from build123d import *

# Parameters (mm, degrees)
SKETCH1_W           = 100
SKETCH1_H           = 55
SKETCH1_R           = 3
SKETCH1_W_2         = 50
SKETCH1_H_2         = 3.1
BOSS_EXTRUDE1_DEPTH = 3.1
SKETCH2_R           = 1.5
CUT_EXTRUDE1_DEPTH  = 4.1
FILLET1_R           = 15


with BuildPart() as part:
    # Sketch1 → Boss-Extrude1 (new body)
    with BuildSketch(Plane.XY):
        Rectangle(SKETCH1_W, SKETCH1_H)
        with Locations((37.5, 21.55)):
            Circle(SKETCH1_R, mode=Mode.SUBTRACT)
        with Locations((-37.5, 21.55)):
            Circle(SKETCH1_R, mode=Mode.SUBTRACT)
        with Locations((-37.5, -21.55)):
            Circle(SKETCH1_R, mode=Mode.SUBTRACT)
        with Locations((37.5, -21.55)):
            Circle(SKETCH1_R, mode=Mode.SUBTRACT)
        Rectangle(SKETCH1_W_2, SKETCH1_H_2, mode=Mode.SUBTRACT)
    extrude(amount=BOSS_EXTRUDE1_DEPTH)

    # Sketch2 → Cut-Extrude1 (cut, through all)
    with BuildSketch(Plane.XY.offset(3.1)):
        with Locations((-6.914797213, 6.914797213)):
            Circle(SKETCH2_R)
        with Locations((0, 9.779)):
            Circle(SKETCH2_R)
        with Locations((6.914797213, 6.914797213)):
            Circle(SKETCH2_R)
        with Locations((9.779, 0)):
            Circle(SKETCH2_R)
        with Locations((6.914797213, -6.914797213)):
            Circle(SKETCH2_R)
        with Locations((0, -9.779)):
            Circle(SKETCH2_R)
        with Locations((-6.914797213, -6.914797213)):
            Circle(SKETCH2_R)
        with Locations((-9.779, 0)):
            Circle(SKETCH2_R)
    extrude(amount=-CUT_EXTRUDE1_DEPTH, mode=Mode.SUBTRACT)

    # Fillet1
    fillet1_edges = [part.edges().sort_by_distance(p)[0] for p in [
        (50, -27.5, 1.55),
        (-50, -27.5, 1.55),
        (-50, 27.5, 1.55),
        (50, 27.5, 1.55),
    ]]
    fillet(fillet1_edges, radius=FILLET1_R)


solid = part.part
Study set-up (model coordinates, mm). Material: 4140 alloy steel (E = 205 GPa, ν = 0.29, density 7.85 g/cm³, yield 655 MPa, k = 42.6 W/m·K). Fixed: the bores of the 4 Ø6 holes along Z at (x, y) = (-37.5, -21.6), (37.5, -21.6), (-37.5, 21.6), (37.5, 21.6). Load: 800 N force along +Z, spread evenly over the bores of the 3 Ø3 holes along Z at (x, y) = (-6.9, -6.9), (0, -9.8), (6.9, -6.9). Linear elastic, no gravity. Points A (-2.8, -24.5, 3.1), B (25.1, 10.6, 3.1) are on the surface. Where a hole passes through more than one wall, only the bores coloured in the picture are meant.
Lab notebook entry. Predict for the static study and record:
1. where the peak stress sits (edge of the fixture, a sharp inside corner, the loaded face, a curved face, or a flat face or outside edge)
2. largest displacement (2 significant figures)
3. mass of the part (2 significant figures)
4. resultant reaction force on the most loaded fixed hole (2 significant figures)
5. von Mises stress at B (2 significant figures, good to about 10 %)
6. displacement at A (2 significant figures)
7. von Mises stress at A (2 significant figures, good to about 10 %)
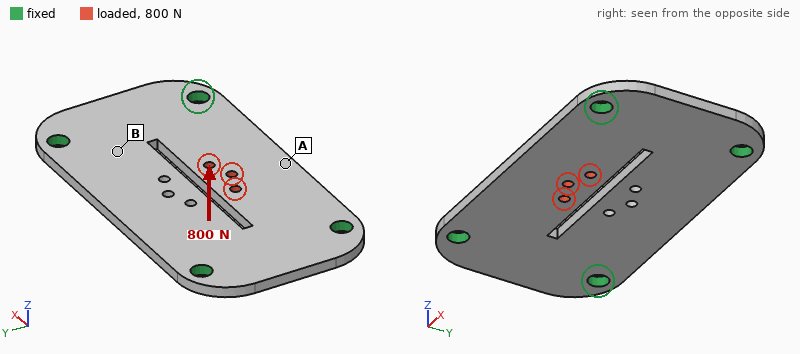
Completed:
the loaded face
0.16 mm
120 g
290 N
28 MPa
0.081 mm
97 MPa
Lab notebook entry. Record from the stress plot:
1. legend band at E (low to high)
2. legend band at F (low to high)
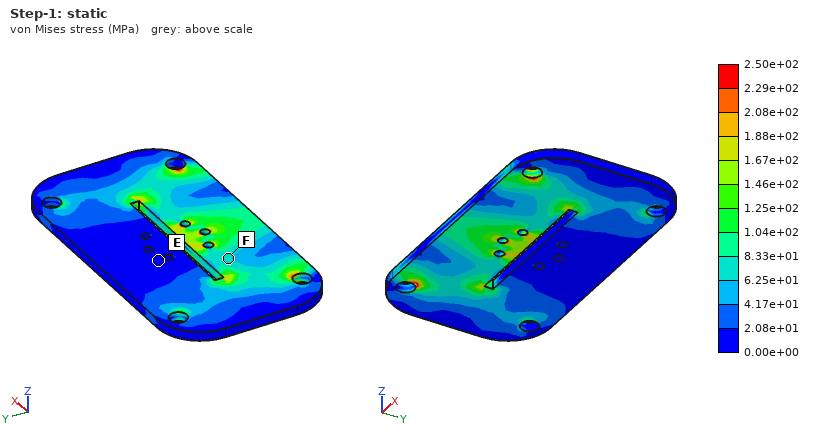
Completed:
0.00e+00 to 2.08e+01 MPa
6.25e+01 to 8.33e+01 MPa
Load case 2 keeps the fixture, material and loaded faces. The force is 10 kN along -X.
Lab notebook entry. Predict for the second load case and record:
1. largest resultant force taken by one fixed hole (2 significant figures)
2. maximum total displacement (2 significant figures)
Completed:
4.2 kN
18 µm
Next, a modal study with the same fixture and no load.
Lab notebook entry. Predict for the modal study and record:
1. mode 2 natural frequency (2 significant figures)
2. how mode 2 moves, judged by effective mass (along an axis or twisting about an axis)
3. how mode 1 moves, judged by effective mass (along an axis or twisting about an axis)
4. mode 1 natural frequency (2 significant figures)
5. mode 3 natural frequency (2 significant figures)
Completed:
3500 Hz
twisting about X
along Z
2800 Hz
5700 Hz
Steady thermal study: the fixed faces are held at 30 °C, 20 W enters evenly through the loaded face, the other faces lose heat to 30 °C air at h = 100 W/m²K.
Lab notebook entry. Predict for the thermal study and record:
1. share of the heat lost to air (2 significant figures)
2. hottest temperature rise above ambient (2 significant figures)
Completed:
64 %
75 K
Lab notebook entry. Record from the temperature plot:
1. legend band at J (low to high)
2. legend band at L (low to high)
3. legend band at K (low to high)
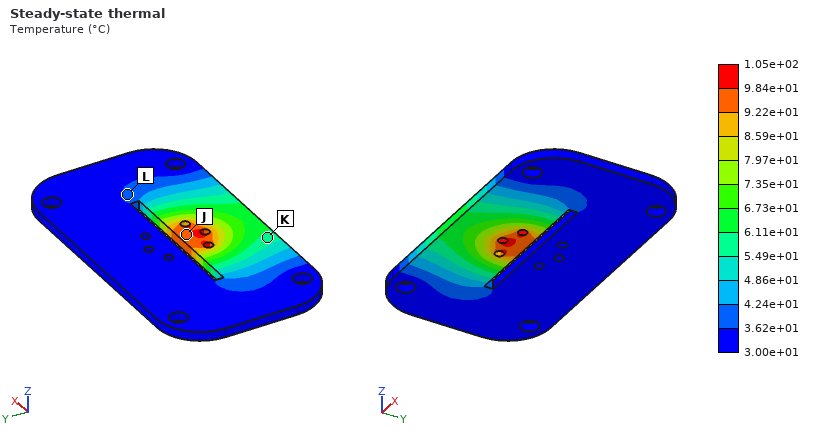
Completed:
9.22e+01 to 9.84e+01 °C
3.62e+01 to 4.24e+01 °C
5.49e+01 to 6.11e+01 °C
